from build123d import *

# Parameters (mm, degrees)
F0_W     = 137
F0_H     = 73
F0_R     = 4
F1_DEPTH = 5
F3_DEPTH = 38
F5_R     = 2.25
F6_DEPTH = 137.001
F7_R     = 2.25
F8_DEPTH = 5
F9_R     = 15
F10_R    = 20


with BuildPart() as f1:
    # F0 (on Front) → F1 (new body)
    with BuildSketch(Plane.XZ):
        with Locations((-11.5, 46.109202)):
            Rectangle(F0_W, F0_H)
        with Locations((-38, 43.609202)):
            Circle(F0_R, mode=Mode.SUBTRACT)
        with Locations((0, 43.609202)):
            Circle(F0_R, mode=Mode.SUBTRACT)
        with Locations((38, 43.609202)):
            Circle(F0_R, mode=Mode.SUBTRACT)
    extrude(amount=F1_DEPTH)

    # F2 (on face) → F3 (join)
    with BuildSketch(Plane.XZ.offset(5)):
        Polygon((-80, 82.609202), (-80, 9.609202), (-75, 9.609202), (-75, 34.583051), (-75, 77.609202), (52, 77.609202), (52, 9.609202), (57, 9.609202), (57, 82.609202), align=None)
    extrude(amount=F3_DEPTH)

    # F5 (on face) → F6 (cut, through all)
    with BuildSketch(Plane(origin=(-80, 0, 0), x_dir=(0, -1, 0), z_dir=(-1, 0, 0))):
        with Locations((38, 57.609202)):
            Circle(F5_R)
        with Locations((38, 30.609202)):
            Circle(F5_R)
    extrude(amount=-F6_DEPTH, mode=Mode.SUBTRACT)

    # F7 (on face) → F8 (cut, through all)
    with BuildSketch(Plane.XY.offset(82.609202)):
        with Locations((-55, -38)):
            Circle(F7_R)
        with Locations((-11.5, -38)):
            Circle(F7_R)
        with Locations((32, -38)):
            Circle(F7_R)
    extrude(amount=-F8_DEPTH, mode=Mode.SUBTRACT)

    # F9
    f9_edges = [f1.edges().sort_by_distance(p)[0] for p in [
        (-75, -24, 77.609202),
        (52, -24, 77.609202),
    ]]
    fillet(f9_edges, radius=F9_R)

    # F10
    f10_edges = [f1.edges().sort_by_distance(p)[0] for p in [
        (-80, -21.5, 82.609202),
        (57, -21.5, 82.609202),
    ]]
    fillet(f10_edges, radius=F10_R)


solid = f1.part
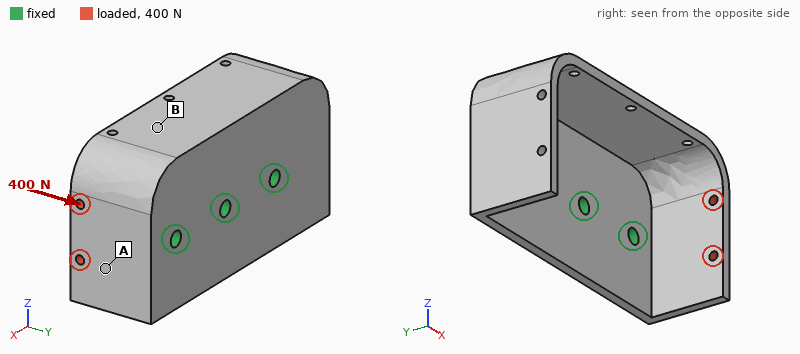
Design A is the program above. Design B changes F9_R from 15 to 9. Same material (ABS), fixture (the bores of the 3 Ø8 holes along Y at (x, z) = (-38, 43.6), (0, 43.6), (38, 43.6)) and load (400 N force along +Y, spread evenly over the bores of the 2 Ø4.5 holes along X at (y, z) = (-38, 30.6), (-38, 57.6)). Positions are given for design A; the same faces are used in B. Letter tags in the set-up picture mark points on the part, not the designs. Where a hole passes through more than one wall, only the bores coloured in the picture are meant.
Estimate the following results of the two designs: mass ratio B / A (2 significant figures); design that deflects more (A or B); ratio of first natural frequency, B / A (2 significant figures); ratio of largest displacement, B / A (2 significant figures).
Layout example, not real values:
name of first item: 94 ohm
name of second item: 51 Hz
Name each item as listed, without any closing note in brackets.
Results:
mass ratio B / A: 0.98
design that deflects more: B
ratio of first natural frequency, B / A: 1.0
ratio of largest displacement, B / A: 1.1
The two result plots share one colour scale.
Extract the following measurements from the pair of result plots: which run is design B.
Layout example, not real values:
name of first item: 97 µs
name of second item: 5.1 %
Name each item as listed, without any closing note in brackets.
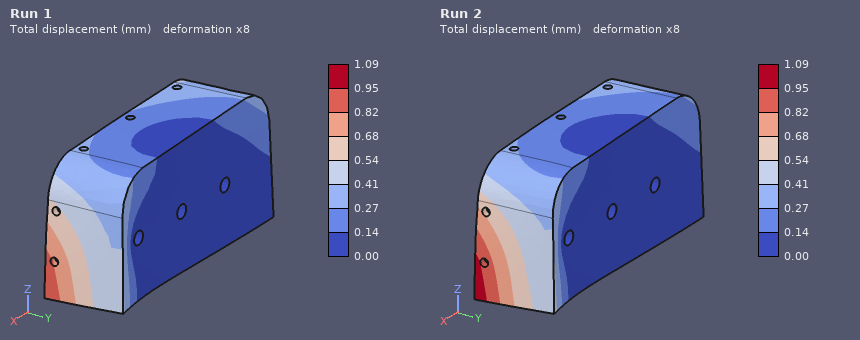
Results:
which run is design B: Run 2
